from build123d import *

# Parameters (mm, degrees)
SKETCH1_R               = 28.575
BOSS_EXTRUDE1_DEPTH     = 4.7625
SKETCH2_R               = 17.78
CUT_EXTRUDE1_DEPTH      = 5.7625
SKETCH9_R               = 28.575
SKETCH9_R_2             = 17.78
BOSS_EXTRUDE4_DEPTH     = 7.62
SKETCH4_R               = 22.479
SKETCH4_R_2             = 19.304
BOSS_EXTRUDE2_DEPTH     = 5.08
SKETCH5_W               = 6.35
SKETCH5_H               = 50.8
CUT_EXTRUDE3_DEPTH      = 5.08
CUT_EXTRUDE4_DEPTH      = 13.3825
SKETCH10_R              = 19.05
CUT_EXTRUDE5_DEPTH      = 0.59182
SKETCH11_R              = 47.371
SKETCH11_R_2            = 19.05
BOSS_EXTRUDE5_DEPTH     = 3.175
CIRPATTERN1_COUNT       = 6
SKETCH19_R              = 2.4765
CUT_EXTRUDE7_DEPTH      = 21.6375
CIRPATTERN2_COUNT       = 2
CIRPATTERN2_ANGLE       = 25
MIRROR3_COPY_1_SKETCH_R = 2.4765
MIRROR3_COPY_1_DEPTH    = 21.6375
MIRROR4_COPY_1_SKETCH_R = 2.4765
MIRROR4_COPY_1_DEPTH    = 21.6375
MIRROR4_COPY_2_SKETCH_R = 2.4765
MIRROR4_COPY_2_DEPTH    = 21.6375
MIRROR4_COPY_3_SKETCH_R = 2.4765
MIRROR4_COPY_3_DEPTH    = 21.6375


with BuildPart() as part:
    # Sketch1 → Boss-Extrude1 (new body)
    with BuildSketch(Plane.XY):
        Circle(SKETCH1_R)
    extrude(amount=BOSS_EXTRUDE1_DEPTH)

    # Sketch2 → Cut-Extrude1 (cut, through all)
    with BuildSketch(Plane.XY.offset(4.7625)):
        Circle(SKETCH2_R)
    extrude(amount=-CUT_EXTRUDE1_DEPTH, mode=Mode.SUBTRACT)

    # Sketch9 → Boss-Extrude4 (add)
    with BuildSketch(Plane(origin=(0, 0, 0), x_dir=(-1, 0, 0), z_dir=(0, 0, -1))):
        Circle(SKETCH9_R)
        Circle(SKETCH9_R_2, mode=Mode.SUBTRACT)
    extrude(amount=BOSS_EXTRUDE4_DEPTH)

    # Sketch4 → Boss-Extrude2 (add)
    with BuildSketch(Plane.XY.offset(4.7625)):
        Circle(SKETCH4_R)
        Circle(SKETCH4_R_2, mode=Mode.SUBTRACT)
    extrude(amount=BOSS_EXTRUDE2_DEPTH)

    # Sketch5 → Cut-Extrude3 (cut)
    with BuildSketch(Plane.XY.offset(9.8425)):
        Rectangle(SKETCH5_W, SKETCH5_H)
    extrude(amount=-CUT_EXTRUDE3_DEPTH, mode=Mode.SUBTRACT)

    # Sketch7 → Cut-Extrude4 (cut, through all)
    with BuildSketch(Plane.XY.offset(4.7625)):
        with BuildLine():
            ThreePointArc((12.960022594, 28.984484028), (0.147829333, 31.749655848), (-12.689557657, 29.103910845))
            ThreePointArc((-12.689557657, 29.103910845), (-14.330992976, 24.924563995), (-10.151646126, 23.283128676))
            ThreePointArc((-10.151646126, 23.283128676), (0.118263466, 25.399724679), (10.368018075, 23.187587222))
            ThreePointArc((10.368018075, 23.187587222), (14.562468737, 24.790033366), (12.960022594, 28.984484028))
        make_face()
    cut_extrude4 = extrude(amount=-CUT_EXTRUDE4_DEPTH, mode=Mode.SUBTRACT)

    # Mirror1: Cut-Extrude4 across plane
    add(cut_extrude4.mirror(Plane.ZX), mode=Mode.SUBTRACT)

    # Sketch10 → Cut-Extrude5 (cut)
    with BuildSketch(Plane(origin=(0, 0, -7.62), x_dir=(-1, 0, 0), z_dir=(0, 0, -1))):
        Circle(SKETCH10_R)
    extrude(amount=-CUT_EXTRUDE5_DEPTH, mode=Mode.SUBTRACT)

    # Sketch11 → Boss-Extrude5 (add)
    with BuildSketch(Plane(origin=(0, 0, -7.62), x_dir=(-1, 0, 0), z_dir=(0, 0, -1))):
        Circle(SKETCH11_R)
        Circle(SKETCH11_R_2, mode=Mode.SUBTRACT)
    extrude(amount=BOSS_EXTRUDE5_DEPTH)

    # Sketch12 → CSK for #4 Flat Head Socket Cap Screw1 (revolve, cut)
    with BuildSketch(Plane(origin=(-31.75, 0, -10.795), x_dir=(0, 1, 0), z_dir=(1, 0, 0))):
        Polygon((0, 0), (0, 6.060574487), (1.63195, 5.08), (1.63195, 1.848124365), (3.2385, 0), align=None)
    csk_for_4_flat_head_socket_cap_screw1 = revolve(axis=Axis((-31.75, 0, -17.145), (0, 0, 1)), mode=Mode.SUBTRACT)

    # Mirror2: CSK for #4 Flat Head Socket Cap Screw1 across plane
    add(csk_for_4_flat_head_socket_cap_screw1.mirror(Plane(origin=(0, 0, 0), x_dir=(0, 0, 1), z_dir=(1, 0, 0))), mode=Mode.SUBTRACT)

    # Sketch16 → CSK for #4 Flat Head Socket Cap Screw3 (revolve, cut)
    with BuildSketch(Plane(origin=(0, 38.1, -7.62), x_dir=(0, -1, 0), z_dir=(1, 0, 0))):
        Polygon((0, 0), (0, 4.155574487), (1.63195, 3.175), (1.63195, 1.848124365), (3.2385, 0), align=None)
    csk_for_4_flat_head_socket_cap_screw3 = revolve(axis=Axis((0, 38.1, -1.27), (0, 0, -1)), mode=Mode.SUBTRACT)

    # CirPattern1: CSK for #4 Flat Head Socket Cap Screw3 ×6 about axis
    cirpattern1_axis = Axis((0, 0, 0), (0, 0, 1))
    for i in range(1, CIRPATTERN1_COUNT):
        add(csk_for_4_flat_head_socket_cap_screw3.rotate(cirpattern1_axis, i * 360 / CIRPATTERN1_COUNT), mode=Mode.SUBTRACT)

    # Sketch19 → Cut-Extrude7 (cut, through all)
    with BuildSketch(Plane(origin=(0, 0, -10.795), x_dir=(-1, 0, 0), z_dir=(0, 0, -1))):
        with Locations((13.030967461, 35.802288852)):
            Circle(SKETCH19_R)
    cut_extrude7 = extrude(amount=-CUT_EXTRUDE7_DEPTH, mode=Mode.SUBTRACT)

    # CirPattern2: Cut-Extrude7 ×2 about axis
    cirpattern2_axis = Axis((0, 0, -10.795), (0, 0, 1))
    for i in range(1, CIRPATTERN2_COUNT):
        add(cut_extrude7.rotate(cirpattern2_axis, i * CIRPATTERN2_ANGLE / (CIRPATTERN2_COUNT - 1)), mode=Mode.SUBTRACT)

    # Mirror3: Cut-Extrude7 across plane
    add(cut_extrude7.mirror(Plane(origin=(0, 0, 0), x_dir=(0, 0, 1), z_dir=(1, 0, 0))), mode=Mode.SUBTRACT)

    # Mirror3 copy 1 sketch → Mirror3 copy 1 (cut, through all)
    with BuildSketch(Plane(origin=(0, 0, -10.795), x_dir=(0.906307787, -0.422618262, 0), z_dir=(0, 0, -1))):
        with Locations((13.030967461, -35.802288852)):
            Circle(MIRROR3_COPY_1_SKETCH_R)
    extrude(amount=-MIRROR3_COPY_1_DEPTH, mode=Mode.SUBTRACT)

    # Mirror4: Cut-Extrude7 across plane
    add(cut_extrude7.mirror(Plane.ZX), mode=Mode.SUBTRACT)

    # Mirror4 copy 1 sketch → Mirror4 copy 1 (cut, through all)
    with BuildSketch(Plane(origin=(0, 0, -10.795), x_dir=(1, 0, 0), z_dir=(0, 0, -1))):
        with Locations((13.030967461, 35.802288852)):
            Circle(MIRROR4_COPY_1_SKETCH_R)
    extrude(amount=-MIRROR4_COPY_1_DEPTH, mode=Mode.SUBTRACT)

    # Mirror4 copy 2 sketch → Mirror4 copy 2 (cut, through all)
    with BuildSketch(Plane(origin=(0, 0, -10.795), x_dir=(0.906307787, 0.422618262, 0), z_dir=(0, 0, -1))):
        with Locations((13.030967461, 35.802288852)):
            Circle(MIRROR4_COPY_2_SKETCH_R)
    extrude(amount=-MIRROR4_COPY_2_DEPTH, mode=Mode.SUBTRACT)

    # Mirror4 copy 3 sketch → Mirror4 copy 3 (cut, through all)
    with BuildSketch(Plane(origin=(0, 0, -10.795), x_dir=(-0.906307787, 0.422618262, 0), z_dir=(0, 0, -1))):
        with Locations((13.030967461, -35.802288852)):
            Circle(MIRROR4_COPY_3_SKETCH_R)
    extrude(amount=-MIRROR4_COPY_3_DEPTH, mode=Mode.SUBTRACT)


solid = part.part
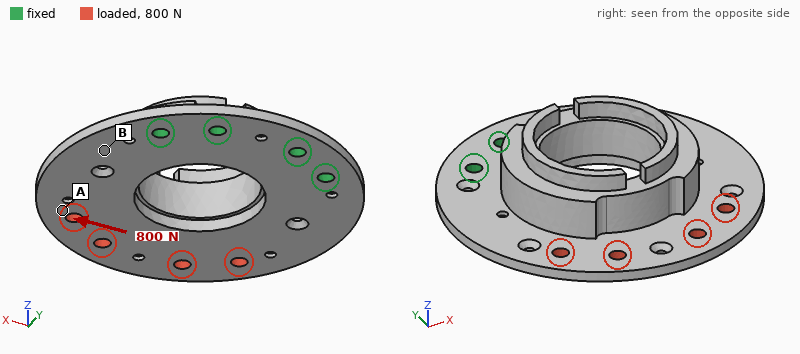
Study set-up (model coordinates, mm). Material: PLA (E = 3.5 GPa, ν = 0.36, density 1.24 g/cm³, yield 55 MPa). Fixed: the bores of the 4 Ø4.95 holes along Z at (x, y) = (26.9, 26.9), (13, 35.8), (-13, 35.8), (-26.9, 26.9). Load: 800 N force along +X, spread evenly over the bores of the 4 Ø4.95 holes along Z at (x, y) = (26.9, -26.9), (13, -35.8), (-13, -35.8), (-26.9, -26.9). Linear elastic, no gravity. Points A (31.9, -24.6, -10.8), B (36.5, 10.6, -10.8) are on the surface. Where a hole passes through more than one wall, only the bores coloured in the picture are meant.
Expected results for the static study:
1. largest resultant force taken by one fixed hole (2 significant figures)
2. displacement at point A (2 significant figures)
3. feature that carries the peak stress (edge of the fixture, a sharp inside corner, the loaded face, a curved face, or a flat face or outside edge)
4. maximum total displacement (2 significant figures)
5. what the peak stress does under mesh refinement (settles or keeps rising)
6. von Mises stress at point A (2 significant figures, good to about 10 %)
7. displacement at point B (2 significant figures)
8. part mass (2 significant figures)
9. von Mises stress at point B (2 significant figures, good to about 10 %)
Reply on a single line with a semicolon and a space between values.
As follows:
890 N; 0.68 mm; edge of the fixture; 0.77 mm; keeps rising; 4.1 MPa; 0.25 mm; 46 g; 8.2 MPa
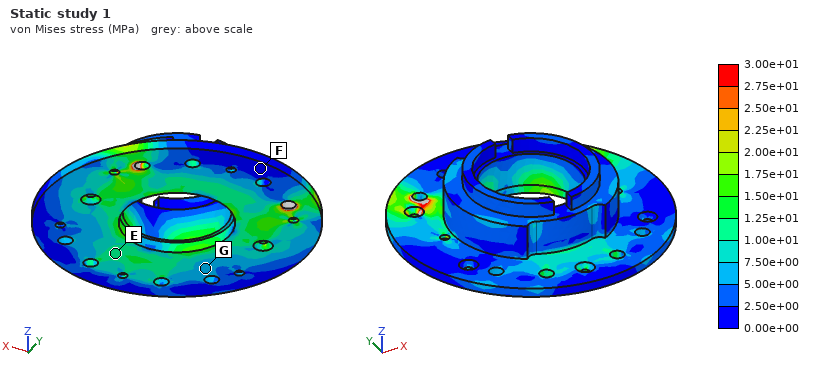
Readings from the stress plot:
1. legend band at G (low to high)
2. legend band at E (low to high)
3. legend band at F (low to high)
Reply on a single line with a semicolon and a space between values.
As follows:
5.00e+00 to 7.50e+00 MPa; 1.00e+01 to 1.25e+01 MPa; 0.00e+00 to 2.50e+00 MPa
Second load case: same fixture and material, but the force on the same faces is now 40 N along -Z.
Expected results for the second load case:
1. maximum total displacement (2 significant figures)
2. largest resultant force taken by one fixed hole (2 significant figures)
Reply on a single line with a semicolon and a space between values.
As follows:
1.6 mm; 93 N
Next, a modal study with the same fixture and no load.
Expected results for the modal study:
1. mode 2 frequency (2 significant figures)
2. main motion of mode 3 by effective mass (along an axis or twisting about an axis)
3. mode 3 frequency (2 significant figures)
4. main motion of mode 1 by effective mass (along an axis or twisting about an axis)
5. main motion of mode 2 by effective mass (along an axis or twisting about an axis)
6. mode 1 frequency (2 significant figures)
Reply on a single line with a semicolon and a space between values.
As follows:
950 Hz; along X; 1500 Hz; along Z; twisting about Y; 240 Hz
